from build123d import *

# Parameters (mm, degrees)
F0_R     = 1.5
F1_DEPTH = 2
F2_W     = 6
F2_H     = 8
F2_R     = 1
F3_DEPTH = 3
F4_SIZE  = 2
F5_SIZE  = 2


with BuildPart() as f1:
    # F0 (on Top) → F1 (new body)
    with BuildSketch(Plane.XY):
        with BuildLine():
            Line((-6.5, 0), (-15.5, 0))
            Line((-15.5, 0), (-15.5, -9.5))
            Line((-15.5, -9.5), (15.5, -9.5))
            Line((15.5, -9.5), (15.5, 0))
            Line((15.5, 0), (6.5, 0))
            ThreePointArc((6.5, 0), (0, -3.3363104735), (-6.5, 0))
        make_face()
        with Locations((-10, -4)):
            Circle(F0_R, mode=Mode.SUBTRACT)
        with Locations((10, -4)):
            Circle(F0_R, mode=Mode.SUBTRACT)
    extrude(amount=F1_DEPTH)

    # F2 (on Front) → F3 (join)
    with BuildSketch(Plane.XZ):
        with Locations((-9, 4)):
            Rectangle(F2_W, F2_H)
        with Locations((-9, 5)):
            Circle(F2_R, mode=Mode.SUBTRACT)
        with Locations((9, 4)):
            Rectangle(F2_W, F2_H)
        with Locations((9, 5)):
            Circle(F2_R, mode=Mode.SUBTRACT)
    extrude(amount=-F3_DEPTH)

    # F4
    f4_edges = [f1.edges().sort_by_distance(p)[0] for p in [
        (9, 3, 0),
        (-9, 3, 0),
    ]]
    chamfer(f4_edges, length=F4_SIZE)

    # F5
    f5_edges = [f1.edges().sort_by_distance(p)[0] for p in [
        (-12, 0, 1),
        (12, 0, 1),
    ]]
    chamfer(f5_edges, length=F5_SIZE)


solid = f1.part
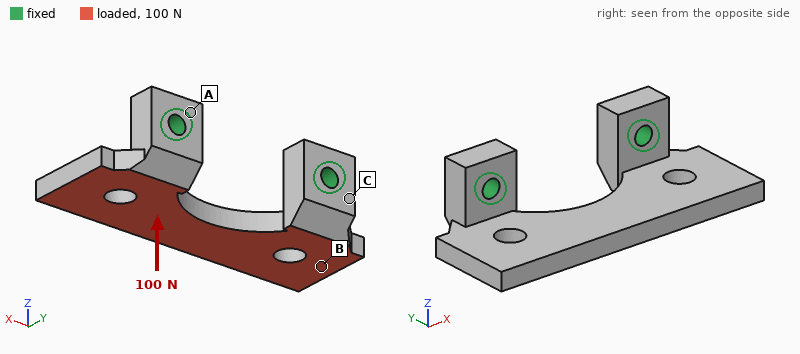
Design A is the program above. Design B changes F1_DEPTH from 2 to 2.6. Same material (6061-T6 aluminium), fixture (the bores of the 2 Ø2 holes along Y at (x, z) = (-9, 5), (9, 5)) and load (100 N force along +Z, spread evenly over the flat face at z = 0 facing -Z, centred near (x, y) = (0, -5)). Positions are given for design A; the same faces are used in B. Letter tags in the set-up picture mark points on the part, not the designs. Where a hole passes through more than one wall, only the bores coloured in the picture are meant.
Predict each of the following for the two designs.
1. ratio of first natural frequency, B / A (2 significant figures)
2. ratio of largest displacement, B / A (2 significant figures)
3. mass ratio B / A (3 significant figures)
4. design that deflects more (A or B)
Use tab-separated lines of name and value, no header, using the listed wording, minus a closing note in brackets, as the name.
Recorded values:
ratio of first natural frequency, B / A	1.1
ratio of largest displacement, B / A	0.62
mass ratio B / A	1.20
design that deflects more	A
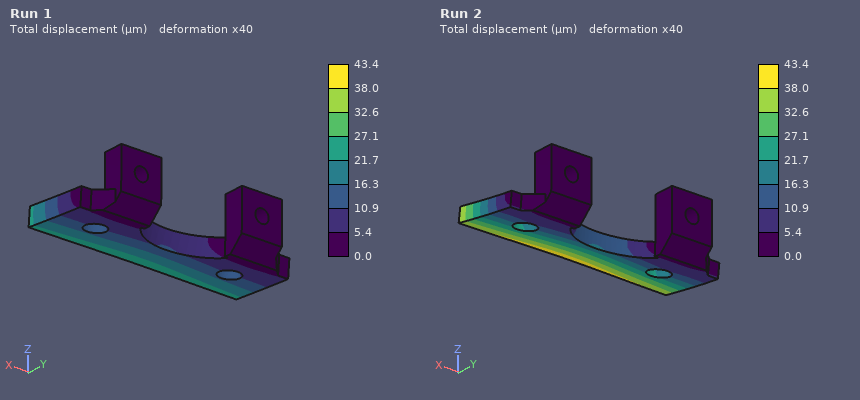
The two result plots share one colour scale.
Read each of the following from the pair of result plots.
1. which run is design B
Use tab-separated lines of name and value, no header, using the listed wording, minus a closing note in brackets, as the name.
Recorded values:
which run is design B	Run 1
